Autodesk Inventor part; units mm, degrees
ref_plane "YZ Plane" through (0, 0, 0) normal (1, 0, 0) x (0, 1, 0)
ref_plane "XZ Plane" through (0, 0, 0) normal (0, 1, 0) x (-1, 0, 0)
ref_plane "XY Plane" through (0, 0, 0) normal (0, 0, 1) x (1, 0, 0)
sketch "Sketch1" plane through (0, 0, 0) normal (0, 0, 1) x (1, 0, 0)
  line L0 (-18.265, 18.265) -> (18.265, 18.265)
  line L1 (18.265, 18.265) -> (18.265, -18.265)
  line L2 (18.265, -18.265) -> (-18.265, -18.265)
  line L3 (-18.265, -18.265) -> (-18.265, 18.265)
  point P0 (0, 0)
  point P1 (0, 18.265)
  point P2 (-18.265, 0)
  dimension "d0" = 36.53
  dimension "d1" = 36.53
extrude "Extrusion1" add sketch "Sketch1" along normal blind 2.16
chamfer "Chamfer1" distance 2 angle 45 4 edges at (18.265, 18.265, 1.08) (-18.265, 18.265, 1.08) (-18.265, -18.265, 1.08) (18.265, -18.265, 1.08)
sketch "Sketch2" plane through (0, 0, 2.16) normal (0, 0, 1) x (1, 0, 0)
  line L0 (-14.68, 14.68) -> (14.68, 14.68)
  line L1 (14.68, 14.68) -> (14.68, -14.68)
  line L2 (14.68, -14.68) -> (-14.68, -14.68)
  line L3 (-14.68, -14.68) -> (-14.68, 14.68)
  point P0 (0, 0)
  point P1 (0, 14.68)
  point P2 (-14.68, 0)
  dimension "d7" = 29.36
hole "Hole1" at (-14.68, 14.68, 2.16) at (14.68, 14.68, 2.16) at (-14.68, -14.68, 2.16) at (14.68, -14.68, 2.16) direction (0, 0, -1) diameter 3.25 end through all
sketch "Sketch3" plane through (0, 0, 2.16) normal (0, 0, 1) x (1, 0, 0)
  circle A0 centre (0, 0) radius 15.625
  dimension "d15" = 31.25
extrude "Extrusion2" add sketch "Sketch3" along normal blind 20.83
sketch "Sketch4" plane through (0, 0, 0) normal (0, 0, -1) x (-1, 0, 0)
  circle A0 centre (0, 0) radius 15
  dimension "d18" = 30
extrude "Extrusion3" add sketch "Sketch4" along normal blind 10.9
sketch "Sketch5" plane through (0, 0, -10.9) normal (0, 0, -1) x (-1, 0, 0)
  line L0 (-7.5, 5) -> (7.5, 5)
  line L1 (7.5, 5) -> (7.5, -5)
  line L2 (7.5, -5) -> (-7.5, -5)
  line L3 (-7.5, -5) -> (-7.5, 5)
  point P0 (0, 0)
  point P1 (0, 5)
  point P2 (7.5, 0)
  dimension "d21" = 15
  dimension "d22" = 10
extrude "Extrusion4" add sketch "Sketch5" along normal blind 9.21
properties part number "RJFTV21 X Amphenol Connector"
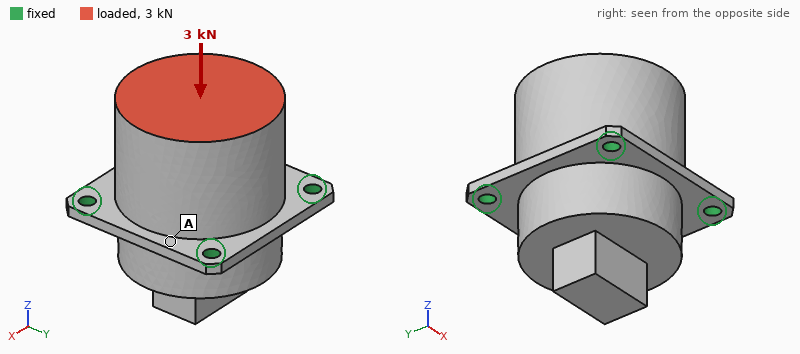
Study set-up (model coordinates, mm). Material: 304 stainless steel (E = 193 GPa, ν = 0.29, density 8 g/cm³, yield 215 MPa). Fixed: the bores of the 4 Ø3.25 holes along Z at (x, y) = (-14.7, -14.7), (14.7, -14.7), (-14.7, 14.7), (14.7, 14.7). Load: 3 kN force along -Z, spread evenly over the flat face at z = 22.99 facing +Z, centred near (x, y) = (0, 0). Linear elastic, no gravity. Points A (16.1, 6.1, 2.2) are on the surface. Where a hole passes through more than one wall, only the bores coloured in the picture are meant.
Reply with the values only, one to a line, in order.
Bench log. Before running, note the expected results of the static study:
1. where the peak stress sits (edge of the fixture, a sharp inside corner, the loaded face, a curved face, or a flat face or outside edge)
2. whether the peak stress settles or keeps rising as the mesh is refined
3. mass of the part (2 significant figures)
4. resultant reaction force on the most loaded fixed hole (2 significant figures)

edge of the fixture
keeps rising
220 g
760 N
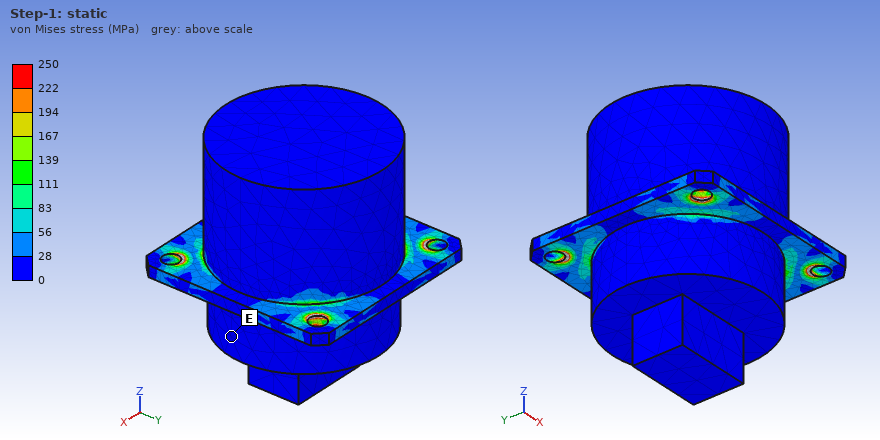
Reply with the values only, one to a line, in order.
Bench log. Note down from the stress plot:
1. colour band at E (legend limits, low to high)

0 to 28 MPa
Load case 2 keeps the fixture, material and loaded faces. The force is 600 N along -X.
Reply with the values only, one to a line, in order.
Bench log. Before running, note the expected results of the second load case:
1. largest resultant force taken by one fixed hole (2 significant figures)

300 N
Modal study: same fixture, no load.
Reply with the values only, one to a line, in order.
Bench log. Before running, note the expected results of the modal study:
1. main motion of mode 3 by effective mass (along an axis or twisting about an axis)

along Z
